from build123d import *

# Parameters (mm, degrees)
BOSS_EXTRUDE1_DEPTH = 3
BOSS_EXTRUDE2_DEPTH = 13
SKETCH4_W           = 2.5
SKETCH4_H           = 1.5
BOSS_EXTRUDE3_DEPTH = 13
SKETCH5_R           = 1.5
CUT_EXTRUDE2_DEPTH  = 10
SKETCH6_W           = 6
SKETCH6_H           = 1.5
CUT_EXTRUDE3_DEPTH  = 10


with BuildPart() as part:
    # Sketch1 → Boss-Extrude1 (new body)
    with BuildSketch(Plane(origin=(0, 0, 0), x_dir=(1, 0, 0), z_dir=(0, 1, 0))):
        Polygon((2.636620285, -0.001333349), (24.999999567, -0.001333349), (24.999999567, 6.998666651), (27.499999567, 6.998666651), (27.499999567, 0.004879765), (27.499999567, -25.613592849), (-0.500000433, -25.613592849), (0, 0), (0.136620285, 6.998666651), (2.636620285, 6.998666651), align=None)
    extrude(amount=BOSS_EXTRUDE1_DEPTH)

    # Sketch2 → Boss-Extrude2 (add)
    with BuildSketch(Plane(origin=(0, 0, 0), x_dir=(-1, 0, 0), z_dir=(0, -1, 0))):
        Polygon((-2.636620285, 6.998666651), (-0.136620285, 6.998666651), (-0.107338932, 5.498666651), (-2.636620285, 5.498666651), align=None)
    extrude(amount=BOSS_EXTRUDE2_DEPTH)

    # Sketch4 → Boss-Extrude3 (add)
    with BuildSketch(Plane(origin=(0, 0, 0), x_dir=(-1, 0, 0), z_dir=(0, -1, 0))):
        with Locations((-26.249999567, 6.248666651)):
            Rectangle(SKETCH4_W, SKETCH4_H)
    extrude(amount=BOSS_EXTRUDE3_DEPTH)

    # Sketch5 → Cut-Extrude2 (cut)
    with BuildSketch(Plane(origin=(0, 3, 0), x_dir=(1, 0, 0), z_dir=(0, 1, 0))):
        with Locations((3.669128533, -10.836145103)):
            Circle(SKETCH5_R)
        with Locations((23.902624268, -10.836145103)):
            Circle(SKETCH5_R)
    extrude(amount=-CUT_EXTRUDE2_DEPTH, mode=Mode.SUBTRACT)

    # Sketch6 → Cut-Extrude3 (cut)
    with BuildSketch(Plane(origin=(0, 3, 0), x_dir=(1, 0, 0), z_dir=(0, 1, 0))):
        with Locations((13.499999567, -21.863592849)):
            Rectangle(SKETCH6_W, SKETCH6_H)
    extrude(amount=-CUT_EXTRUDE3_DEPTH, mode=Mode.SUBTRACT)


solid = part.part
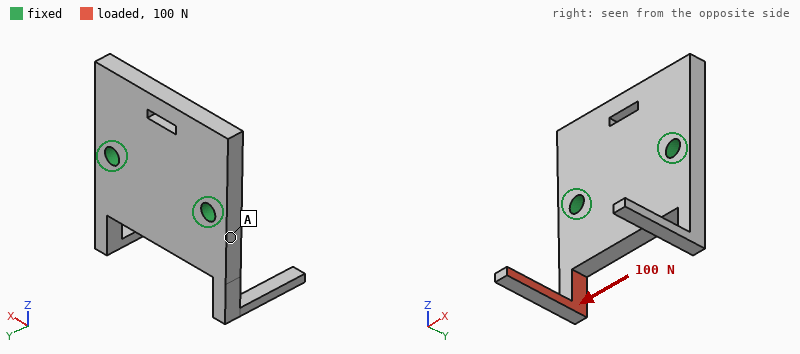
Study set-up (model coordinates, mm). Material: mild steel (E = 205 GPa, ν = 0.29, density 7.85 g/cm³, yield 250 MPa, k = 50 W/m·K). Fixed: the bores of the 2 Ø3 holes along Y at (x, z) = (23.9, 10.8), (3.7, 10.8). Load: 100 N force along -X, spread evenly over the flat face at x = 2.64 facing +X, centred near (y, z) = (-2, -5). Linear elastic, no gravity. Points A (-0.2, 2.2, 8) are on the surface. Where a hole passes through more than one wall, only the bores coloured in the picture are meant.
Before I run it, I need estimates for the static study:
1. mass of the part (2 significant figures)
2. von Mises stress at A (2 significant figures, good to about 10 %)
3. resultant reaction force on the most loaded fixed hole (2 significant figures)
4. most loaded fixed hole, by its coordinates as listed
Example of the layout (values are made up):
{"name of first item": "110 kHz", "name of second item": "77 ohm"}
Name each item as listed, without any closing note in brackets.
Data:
{"mass of the part": "18 g", "von Mises stress at A": "19 MPa", "resultant reaction force on the most loaded fixed hole": "97 N", "most loaded fixed hole, by its coordinates as listed": "(23.9, 10.8)"}
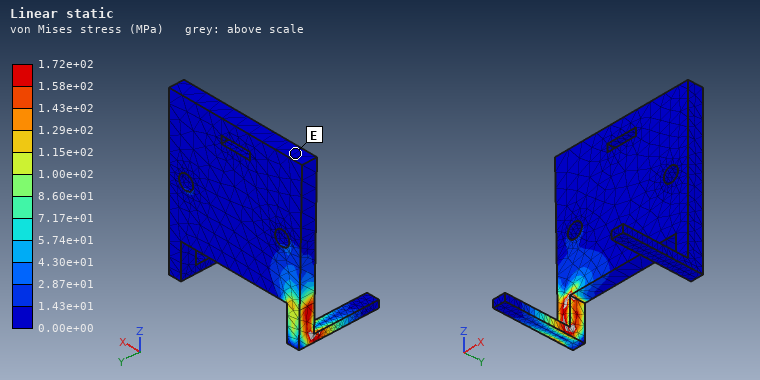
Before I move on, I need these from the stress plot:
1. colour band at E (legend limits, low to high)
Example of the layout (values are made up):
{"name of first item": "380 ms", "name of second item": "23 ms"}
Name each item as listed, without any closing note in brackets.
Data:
{"colour band at E": "0.00e+00 to 1.43e+01 MPa"}
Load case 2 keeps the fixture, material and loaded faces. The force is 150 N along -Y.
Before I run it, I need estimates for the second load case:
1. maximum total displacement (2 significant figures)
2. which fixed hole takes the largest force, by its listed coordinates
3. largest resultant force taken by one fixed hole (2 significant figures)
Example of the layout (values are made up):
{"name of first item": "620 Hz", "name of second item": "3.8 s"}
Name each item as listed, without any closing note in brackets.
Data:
{"maximum total displacement": "0.11 mm", "which fixed hole takes the largest force, by its listed coordinates": "(3.7, 10.8)", "largest resultant force taken by one fixed hole": "160 N"}
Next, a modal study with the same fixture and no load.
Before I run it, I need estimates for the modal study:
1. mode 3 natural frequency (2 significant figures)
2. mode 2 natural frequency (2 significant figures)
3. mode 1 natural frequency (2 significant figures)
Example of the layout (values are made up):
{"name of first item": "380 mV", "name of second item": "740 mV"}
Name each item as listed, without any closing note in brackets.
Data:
{"mode 3 natural frequency": "6100 Hz", "mode 2 natural frequency": "5300 Hz", "mode 1 natural frequency": "5200 Hz"}
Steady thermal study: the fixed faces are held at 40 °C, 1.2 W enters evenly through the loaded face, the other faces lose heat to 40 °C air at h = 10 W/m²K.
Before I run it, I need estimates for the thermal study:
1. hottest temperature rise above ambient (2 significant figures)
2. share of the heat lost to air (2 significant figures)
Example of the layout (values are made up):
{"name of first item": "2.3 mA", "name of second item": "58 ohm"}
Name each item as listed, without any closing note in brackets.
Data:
{"hottest temperature rise above ambient": "46 K", "share of the heat lost to air": "5.5 %"}
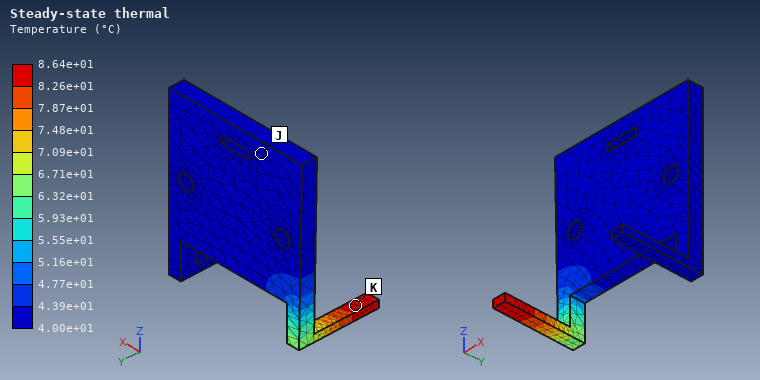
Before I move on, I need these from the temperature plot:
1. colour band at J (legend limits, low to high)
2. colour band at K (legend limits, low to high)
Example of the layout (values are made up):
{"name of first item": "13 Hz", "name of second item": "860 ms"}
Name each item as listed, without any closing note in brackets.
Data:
{"colour band at J": "4.00e+01 to 4.39e+01 °C", "colour band at K": "8.26e+01 to 8.64e+01 °C"}
